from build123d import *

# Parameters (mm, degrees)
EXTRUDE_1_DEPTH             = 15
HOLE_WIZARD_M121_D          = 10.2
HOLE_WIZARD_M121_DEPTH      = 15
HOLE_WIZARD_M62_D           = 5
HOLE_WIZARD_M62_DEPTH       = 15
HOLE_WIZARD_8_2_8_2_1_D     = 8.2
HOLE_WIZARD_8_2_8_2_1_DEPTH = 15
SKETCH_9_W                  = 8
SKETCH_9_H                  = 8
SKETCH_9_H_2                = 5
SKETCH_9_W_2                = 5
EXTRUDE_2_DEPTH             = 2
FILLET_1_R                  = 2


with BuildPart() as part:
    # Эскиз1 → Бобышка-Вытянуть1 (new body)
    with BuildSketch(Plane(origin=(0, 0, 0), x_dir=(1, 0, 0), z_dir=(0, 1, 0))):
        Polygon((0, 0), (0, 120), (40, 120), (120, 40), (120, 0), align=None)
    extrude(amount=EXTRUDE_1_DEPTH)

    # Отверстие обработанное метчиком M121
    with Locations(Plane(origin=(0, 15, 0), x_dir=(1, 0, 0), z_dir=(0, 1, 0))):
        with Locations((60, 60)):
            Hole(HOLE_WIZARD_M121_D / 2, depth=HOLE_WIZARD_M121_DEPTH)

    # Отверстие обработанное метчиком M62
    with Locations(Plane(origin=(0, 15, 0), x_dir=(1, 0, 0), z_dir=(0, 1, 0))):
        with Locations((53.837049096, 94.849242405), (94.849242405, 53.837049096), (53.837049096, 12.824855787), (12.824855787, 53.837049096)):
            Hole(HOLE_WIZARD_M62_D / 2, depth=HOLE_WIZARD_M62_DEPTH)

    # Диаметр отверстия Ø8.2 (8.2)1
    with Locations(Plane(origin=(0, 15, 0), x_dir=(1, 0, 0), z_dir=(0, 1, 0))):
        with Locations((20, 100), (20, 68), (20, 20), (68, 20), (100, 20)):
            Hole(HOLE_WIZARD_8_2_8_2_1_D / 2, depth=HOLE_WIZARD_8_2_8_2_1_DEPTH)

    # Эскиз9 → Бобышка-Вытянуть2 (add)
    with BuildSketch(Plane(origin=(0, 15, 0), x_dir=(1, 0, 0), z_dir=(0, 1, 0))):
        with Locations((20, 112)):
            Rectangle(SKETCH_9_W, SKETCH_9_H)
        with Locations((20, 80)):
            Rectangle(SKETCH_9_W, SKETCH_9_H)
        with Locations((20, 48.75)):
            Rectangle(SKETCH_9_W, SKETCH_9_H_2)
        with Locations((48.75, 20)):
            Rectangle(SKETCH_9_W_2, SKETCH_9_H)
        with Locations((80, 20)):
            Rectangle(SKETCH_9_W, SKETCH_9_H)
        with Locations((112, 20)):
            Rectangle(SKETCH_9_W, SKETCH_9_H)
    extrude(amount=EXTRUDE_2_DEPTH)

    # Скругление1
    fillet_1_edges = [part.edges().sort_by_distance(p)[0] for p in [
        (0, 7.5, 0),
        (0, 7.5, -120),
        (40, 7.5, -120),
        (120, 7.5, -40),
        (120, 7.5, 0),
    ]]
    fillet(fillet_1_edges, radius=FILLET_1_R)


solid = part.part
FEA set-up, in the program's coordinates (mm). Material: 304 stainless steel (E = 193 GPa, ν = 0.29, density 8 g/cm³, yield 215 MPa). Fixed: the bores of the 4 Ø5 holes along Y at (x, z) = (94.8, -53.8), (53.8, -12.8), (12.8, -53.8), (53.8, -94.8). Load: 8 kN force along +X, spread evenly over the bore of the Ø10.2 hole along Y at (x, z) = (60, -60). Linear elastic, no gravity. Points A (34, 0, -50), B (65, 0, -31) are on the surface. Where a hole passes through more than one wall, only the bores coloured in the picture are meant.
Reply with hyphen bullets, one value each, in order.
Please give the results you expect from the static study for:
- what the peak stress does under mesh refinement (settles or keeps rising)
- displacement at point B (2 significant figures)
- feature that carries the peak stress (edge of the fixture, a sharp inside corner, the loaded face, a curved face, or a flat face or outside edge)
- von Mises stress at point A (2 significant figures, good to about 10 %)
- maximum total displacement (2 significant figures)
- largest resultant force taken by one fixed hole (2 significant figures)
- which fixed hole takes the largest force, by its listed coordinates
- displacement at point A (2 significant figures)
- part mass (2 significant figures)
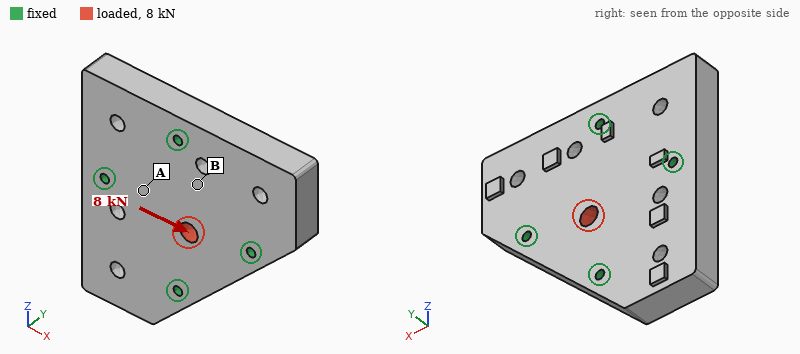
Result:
- keeps rising
- 0.50 µm
- edge of the fixture
- 6.5 MPa
- 2.2 µm
- 3.0 kN
- (94.8, -53.8)
- 0.80 µm
- 1.3 kg
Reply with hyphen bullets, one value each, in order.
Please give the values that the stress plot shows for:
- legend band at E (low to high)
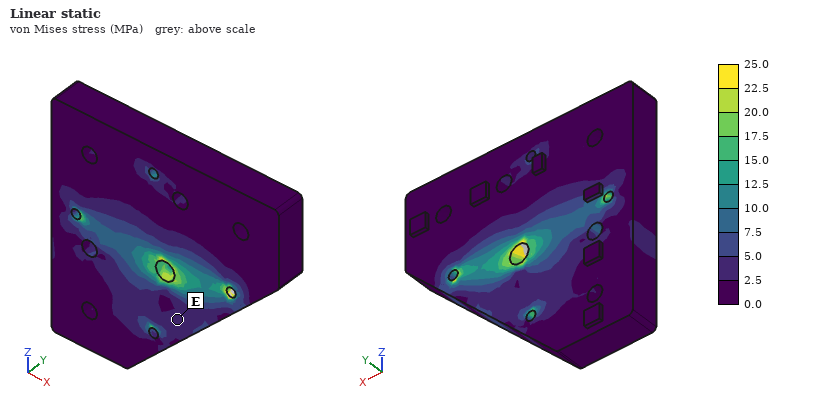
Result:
- 2.5 to 5.0 MPa
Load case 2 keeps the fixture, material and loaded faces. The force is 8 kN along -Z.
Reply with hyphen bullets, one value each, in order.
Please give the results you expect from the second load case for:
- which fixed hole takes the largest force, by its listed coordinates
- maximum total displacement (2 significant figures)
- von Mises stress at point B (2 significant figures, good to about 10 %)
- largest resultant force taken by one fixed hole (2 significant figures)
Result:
- (53.8, -94.8)
- 2.2 µm
- 6.1 MPa
- 3.0 kN
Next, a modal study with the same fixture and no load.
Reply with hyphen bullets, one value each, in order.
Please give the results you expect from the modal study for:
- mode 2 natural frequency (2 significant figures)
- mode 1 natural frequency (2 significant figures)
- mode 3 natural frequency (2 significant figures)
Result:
- 4900 Hz
- 4800 Hz
- 6700 Hz
